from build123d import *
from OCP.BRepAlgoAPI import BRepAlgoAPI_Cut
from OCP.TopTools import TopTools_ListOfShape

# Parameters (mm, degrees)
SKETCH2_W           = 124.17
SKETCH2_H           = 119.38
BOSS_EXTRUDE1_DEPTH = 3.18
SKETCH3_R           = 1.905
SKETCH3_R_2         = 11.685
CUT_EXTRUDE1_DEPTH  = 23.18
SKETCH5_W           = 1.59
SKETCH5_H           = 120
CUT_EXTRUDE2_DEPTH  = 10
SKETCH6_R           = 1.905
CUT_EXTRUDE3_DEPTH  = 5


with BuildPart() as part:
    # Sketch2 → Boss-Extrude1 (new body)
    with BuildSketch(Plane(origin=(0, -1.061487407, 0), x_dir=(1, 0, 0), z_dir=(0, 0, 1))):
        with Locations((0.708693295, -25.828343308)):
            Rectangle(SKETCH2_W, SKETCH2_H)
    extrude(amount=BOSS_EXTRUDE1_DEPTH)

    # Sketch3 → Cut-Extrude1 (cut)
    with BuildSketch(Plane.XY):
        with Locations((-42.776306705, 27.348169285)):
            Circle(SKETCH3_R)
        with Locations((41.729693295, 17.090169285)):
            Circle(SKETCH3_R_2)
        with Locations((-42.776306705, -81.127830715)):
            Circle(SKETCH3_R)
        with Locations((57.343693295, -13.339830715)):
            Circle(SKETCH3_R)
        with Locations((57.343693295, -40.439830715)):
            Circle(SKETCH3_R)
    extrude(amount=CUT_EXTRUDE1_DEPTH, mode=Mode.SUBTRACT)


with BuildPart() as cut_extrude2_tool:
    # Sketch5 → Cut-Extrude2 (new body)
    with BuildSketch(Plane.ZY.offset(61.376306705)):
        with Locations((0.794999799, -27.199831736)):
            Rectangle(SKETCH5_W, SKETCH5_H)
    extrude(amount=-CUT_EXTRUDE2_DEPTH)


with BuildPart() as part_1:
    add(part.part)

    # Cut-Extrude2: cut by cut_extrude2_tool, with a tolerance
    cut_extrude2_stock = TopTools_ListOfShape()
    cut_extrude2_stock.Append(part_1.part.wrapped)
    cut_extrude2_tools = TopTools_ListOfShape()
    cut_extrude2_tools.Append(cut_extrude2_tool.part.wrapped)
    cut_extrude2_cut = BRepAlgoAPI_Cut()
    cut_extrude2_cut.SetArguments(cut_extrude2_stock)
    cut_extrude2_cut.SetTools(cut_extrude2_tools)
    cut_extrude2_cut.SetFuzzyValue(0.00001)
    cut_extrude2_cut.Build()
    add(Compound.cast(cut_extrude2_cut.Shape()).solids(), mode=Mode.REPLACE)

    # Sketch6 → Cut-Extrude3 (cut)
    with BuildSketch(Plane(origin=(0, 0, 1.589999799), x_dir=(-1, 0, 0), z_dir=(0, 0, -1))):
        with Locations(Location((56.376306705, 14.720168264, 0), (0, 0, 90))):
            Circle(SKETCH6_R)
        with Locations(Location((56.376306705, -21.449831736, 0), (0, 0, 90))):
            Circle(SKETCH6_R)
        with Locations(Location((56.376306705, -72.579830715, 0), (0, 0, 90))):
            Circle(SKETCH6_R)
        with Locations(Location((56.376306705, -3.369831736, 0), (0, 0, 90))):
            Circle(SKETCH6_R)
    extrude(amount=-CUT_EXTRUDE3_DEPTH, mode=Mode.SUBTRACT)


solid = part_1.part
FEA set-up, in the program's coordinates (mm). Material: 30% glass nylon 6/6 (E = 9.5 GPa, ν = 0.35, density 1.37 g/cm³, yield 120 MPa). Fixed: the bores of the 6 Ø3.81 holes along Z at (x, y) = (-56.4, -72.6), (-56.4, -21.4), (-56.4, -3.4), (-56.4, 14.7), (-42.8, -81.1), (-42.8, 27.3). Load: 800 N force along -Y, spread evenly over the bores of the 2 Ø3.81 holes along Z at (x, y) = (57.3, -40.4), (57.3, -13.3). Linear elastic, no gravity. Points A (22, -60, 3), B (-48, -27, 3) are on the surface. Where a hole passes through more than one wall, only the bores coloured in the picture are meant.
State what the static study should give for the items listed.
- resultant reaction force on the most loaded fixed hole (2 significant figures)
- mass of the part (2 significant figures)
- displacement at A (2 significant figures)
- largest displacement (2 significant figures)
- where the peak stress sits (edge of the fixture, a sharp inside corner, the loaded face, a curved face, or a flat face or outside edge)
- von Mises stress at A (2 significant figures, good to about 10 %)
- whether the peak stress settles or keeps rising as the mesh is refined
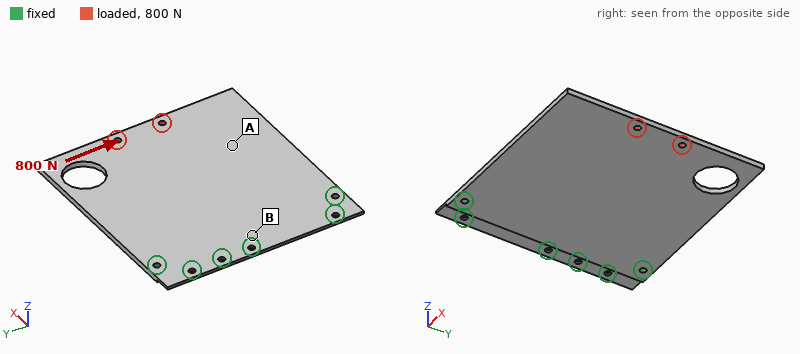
690 N
60 g
0.094 mm
0.17 mm
edge of the fixture
4.9 MPa
keeps rising
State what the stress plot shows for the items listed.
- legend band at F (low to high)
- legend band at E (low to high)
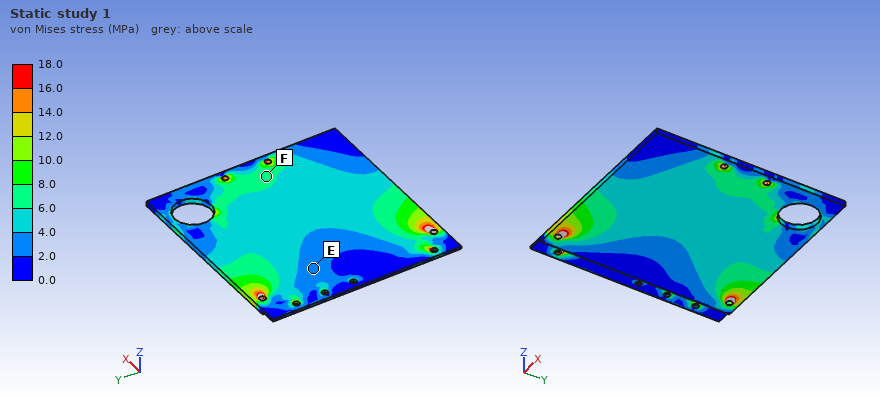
6.0 to 8.0 MPa
2.0 to 4.0 MPa
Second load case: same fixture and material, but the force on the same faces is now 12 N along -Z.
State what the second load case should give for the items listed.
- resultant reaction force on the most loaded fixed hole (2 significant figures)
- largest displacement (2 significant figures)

36 N
2.0 mm
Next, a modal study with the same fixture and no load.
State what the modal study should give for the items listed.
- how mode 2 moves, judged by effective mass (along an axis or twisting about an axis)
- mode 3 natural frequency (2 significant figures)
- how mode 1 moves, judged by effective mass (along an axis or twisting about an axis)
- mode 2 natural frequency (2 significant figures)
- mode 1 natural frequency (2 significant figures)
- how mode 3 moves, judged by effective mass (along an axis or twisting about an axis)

twisting about X
640 Hz
along Z
280 Hz
100 Hz
along Z
